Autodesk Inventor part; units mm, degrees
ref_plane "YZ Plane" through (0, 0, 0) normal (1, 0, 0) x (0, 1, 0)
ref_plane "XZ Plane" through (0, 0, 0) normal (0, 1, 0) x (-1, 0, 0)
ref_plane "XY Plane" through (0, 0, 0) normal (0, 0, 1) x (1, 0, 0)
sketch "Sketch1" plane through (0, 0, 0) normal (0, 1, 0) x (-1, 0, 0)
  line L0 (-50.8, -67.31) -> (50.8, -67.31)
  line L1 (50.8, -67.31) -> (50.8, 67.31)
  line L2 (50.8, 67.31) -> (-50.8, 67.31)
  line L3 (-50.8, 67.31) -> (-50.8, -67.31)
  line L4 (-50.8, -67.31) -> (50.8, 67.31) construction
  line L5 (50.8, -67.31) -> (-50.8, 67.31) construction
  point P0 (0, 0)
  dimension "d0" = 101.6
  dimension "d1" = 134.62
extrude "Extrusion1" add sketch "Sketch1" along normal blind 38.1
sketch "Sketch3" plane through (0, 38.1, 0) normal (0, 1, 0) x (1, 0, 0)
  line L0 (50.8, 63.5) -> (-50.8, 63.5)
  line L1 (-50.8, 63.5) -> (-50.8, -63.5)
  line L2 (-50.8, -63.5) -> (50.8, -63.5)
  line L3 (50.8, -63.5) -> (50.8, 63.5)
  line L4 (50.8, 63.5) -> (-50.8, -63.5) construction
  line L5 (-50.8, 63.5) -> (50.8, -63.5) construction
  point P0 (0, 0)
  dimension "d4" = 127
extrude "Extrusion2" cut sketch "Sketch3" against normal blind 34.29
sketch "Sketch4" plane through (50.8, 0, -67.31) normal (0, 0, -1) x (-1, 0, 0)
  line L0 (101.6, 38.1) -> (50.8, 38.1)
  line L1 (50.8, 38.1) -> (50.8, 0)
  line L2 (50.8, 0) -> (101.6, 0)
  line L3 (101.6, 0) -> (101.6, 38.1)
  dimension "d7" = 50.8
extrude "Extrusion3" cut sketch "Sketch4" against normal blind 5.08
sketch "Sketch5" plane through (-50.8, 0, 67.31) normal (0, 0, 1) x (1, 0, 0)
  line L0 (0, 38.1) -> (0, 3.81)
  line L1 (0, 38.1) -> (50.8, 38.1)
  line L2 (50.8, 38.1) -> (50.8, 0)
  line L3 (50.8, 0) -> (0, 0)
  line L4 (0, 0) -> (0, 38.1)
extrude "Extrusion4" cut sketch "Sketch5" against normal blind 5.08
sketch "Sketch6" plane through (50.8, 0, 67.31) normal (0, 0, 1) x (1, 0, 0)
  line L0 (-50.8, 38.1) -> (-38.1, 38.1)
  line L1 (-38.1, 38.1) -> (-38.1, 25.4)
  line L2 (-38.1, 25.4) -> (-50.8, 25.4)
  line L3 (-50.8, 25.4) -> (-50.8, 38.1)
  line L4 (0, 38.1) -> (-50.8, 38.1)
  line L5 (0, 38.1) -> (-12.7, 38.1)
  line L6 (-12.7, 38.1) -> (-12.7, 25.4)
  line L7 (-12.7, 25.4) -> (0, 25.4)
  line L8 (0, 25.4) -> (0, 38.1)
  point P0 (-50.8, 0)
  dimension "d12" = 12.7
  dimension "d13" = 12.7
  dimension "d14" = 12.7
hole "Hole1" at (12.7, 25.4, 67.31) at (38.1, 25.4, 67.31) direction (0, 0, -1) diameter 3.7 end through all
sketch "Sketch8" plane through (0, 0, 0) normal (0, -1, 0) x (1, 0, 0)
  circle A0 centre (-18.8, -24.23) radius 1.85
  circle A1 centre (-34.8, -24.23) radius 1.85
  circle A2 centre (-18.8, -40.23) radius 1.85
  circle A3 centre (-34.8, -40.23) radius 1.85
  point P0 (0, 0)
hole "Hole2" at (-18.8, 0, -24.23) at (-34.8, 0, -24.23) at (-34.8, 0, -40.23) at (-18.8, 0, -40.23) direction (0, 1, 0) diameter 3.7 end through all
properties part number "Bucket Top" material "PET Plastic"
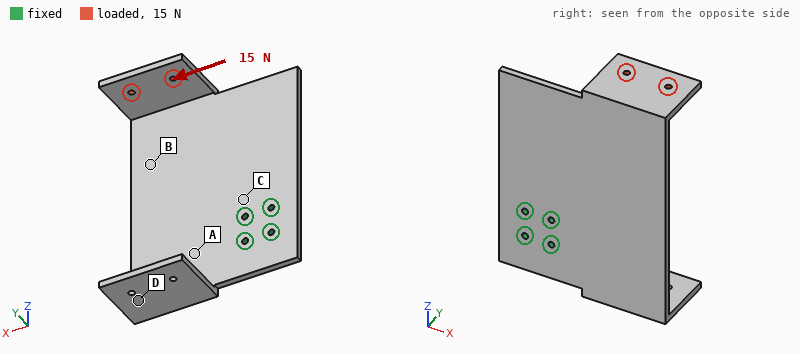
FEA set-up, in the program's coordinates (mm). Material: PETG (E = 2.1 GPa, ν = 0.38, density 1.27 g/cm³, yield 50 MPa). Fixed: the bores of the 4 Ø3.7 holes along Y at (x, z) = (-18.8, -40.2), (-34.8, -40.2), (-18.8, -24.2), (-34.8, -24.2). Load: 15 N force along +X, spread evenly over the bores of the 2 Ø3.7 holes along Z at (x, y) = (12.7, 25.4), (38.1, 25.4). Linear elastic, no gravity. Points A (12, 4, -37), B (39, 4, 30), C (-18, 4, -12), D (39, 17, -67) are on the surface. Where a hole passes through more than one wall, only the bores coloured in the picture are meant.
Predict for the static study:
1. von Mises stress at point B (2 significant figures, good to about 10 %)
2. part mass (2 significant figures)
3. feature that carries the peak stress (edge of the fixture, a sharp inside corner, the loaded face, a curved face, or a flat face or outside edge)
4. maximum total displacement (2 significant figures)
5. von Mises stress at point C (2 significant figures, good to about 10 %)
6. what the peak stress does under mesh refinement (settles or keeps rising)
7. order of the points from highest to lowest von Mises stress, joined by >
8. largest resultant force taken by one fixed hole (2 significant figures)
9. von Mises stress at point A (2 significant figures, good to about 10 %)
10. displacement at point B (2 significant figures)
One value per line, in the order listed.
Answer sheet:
1.4 MPa
80 g
a sharp inside corner
2.0 mm
1.8 MPa
keeps rising
C > B > A > D
38 N
0.64 MPa
0.94 mm
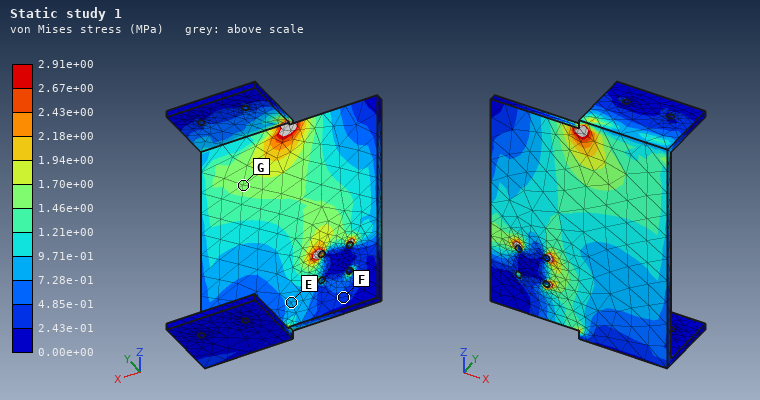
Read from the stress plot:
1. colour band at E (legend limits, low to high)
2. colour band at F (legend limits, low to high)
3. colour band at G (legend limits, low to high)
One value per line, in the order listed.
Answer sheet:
7.28e-01 to 9.71e-01 MPa
2.43e-01 to 4.85e-01 MPa
1.46e+00 to 1.70e+00 MPa
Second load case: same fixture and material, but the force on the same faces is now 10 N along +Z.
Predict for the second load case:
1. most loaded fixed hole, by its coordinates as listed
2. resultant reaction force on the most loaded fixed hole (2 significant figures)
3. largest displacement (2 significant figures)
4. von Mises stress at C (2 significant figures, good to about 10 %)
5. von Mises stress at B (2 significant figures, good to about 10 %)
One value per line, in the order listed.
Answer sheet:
(-18.8, -24.2)
16 N
1.8 mm
1.2 MPa
1.2 MPa
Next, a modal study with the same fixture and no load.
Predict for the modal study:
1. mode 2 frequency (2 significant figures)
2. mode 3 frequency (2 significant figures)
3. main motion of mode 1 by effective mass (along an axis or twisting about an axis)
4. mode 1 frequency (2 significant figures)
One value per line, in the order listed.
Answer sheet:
110 Hz
160 Hz
along Y
58 Hz
